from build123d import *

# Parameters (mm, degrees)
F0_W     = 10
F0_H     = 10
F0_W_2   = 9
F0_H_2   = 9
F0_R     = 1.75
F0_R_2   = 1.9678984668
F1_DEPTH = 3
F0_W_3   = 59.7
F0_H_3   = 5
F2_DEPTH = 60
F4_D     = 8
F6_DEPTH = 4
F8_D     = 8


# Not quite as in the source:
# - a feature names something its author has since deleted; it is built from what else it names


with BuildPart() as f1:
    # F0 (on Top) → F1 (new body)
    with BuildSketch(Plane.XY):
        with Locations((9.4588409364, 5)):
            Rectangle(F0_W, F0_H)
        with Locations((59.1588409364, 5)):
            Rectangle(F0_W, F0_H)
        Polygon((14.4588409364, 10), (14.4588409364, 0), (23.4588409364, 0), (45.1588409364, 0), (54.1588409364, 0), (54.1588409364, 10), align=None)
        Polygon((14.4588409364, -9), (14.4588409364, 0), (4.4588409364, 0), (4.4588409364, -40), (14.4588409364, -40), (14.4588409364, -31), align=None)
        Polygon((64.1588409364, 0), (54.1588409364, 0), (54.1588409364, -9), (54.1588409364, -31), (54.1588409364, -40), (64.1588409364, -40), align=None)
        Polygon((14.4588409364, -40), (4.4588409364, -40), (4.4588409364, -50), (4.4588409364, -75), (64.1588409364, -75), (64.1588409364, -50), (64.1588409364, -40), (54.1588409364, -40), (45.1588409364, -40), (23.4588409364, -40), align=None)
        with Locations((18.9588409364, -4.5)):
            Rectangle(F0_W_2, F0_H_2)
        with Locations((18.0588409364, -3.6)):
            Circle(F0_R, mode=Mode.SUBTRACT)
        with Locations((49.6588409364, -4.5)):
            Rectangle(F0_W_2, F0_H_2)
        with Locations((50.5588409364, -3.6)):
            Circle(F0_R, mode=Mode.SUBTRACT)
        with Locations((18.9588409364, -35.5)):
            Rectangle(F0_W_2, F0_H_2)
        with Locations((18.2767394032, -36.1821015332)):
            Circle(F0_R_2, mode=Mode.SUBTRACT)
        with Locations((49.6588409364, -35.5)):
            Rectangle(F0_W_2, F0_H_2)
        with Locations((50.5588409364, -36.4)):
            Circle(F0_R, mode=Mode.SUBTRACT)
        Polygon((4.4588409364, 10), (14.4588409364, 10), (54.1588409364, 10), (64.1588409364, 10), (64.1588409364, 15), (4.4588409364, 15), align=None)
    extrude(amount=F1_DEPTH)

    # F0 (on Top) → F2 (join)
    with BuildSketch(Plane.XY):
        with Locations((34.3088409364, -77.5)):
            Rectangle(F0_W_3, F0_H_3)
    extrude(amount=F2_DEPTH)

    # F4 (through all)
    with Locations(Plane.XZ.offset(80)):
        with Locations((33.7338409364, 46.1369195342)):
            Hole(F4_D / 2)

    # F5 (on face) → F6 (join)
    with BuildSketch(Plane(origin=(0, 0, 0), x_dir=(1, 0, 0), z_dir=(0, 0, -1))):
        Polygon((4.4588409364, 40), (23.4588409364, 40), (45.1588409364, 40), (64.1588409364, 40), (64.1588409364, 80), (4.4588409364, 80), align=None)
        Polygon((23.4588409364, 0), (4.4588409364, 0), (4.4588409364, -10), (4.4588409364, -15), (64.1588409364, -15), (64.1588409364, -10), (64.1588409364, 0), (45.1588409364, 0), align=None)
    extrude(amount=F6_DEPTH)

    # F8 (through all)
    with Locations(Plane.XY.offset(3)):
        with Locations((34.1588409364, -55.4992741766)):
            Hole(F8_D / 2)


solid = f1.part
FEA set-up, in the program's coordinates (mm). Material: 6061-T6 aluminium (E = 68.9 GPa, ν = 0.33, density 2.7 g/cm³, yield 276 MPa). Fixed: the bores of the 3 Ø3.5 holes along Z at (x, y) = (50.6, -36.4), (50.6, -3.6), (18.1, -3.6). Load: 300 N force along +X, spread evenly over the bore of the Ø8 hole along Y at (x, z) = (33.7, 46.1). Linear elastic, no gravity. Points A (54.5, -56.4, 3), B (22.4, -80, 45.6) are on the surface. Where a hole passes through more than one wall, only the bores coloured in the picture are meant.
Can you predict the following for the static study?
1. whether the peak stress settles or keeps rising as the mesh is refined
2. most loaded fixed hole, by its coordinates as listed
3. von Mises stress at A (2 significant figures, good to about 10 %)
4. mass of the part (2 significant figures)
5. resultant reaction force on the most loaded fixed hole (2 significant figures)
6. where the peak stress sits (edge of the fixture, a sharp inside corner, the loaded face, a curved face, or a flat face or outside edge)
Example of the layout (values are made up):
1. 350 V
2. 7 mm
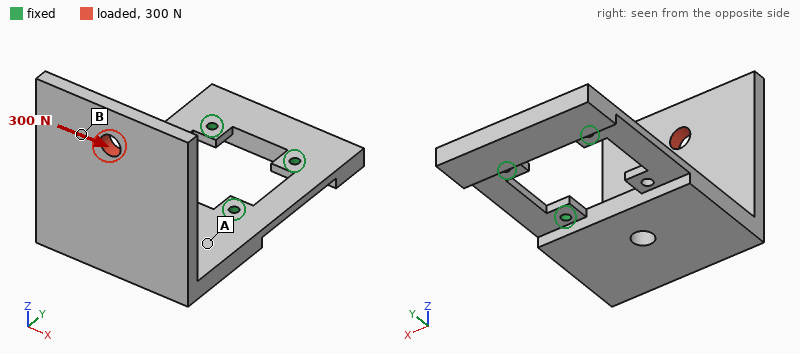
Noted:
1. keeps rising
2. (50.6, -36.4)
3. 45 MPa
4. 120 g
5. 420 N
6. edge of the fixture
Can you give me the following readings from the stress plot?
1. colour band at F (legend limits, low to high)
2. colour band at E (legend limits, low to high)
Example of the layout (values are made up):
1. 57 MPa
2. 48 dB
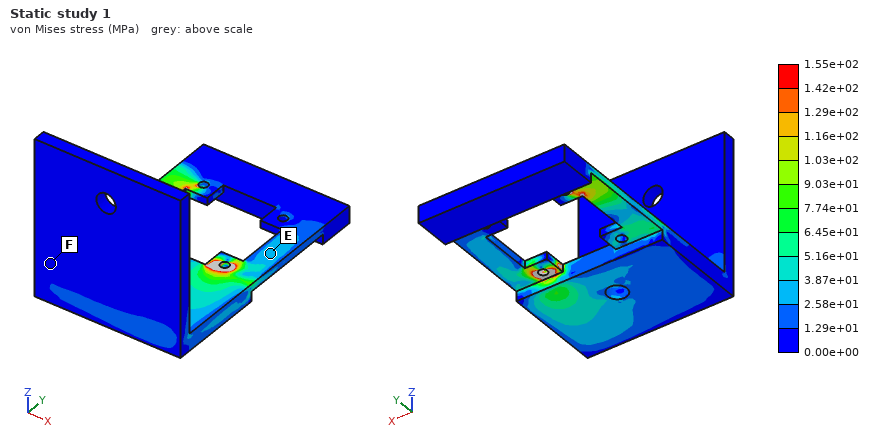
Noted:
1. 0.00e+00 to 1.29e+01 MPa
2. 2.58e+01 to 3.87e+01 MPa
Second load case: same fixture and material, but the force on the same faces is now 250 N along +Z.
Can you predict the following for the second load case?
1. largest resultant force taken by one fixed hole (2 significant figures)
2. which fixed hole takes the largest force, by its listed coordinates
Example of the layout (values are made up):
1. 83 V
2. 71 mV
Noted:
1. 320 N
2. (50.6, -36.4)
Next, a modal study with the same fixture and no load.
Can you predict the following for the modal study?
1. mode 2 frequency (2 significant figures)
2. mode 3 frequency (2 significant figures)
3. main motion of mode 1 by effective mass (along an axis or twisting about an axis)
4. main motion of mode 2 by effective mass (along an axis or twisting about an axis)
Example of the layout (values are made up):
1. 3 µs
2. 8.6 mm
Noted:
1. 580 Hz
2. 1300 Hz
3. along Z
4. along X
